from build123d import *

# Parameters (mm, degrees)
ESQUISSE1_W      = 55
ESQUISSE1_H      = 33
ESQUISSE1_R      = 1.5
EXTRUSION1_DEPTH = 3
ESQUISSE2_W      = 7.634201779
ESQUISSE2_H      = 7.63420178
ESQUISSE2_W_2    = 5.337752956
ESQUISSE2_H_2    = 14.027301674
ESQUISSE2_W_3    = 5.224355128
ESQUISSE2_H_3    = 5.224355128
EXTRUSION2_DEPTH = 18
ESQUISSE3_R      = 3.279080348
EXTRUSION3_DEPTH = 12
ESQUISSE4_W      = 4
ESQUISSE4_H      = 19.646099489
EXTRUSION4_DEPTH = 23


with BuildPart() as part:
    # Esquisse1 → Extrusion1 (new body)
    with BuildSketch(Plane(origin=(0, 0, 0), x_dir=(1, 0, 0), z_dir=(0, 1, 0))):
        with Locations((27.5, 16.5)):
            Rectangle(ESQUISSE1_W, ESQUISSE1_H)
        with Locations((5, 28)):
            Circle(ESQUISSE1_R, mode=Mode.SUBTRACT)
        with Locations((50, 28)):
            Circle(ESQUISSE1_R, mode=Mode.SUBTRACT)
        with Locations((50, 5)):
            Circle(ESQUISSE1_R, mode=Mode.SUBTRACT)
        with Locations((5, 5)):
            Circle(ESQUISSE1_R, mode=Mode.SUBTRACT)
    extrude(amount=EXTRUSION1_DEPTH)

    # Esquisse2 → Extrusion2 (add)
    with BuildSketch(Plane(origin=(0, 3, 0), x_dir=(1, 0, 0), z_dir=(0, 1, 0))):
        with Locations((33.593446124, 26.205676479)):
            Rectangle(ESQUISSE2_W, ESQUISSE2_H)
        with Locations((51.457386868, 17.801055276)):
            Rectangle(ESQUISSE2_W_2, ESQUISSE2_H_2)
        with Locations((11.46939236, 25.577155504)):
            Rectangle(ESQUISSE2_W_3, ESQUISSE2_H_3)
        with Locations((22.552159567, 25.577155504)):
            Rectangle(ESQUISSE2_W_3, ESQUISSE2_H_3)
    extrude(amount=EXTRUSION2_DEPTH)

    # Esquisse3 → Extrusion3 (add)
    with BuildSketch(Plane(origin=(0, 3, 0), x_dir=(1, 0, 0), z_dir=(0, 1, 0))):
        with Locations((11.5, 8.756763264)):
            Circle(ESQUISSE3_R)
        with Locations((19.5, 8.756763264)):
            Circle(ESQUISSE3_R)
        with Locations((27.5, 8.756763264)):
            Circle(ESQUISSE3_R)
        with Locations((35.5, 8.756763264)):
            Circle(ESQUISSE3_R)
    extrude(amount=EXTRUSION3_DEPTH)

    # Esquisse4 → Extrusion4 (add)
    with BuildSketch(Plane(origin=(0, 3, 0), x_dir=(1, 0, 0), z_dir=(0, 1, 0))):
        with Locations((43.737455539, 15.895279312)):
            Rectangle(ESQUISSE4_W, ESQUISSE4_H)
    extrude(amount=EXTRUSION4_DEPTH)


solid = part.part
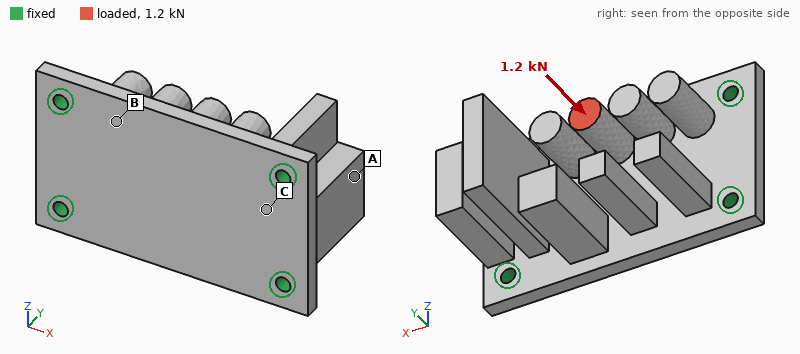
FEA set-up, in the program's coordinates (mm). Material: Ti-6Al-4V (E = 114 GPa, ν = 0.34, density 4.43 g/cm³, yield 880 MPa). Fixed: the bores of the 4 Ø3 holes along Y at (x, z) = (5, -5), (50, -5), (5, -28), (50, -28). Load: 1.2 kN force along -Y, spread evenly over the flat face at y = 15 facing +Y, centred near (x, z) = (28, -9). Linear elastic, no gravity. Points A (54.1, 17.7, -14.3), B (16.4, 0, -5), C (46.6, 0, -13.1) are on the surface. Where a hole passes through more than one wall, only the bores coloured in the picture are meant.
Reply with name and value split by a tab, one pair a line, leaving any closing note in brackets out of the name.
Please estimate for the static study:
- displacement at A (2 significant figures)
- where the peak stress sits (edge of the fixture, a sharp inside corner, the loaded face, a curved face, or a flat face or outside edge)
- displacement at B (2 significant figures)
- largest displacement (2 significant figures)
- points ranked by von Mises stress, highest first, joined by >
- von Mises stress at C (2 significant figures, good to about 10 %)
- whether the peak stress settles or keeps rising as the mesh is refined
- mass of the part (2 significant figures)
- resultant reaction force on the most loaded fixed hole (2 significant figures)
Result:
displacement at A	0.023 mm
where the peak stress sits	edge of the fixture
displacement at B	0.049 mm
largest displacement	0.10 mm
points ranked by von Mises stress, highest first, joined by >	C > B > A
von Mises stress at C	64 MPa
whether the peak stress settles or keeps rising as the mesh is refined	keeps rising
mass of the part	54 g
resultant reaction force on the most loaded fixed hole	520 N
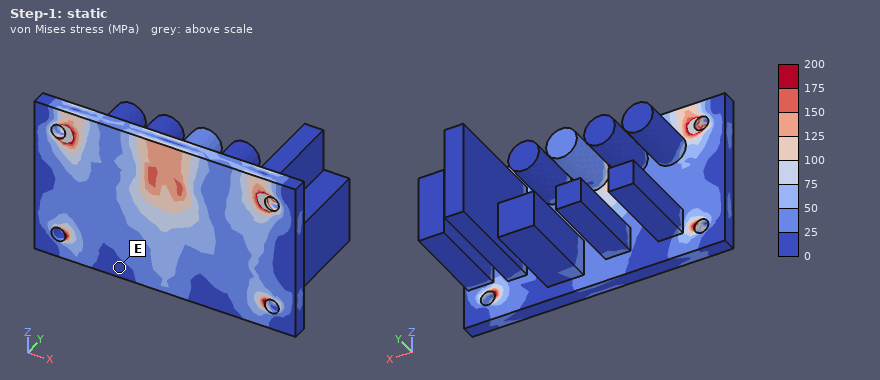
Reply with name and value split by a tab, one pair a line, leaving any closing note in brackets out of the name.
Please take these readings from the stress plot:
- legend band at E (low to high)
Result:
legend band at E	0 to 25 MPa
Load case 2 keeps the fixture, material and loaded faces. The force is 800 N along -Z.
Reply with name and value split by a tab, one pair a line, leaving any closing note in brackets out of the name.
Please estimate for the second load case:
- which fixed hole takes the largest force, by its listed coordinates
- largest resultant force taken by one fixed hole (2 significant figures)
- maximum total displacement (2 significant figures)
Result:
which fixed hole takes the largest force, by its listed coordinates	(50, -28)
largest resultant force taken by one fixed hole	410 N
maximum total displacement	0.17 mm
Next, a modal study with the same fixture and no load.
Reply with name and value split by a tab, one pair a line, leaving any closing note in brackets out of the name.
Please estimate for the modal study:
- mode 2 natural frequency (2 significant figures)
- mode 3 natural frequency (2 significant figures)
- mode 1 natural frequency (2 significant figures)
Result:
mode 2 natural frequency	5100 Hz
mode 3 natural frequency	6000 Hz
mode 1 natural frequency	3700 Hz
